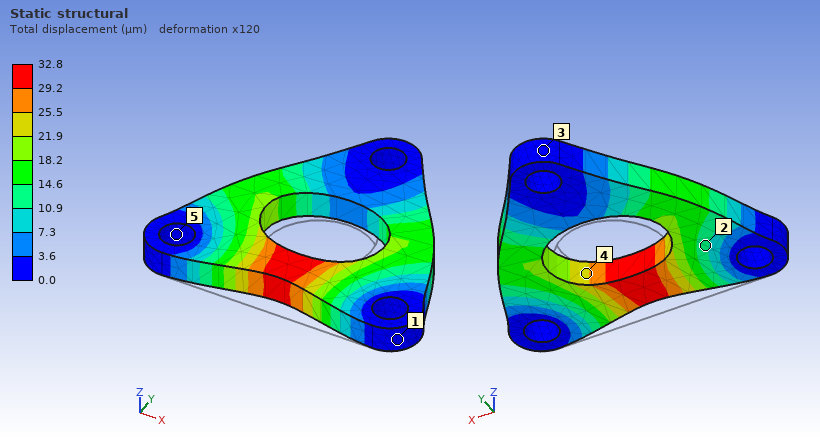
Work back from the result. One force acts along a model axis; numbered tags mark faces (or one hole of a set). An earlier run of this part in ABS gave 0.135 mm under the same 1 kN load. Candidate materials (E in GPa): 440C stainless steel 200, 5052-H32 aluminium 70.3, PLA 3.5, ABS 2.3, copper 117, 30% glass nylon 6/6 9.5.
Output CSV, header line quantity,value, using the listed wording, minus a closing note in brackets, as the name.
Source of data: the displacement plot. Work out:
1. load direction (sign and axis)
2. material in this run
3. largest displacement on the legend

quantity,value
load direction,+Y
material in this run,30% glass nylon 6/6
largest displacement on the legend,32.8 µm
